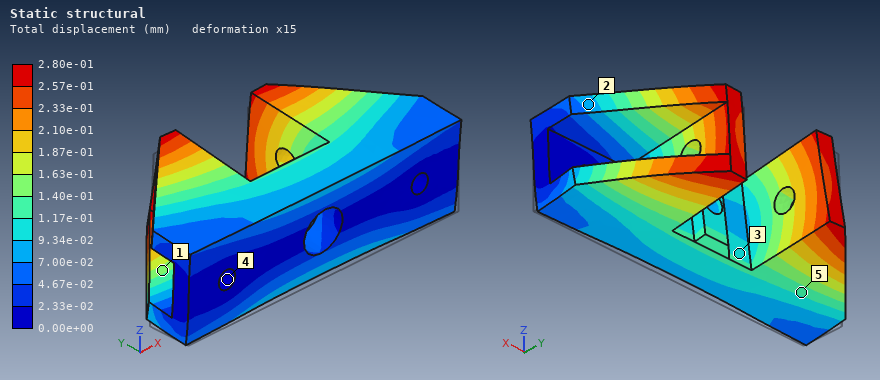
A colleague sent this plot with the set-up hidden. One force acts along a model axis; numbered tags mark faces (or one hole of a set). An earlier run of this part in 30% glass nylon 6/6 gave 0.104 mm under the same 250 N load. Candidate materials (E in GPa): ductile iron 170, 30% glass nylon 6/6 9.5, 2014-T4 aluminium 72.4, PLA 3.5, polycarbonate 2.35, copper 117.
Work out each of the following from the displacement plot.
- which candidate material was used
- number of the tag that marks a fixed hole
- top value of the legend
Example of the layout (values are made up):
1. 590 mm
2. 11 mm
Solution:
1. PLA
2. 4
3. 2.80e-01 mm
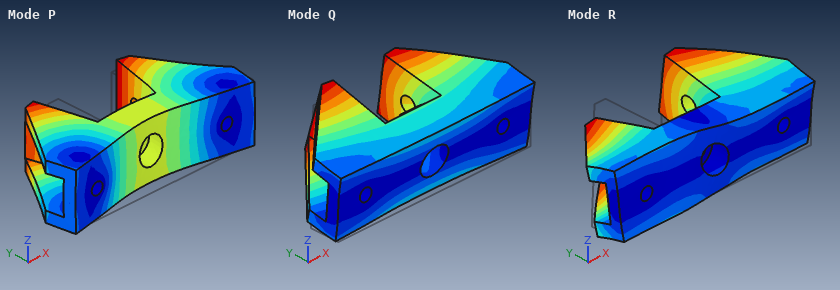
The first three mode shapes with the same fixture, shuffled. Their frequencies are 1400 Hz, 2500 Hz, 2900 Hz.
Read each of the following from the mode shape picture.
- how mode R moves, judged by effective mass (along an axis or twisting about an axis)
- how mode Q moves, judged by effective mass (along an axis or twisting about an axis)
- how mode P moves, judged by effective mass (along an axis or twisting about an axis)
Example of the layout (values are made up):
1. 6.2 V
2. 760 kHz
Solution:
1. twisting about Y
2. along Z
3. along Y
